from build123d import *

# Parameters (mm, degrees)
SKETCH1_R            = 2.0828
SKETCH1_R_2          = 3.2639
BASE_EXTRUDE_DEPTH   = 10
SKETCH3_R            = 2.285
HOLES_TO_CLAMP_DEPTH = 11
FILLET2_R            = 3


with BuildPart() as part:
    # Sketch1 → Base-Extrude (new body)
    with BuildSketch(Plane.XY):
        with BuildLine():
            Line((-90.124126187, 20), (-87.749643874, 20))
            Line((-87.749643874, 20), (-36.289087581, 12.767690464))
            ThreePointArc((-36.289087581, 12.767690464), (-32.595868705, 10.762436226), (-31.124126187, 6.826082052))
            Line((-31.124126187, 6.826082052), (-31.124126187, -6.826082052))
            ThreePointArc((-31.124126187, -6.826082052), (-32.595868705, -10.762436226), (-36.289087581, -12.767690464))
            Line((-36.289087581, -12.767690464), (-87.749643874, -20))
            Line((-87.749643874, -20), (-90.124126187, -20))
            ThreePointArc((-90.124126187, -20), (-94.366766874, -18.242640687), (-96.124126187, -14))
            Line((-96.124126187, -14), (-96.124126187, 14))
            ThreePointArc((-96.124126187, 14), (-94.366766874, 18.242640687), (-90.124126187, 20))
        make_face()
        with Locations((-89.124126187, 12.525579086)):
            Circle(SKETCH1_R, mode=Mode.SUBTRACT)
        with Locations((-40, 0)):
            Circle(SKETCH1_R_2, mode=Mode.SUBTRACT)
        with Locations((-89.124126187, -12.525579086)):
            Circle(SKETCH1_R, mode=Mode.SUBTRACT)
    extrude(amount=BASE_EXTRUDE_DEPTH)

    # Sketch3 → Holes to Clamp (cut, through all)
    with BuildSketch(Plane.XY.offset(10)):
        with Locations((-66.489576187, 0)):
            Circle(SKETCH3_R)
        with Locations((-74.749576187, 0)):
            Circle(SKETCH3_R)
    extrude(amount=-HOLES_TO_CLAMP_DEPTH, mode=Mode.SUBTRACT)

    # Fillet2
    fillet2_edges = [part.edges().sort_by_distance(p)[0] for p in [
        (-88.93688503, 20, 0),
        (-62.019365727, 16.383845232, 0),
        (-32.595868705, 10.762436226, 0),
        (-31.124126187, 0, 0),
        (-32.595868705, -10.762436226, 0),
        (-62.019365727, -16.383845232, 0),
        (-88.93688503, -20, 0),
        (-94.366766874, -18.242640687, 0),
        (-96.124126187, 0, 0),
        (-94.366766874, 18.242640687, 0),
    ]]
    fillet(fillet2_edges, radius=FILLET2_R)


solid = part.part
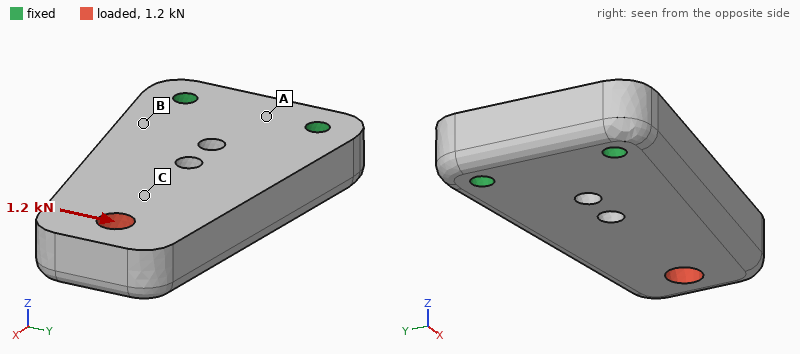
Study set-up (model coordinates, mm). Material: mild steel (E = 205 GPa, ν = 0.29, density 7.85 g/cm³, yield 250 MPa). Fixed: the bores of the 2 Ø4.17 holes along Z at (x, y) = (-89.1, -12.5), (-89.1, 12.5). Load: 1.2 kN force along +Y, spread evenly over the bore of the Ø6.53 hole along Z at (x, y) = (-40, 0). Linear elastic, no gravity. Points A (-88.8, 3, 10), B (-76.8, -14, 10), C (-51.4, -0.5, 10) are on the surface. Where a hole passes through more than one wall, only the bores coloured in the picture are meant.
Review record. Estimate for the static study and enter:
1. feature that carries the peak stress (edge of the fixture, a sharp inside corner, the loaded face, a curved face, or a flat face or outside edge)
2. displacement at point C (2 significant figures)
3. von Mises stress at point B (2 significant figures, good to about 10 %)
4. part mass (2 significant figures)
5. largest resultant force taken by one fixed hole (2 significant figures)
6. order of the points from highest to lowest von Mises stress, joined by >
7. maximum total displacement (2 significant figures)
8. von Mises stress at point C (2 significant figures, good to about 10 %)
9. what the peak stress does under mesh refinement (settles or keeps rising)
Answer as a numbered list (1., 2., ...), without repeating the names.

1. edge of the fixture
2. 6.0 µm
3. 16 MPa
4. 160 g
5. 2.2 kN
6. B > C > A
7. 11 µm
8. 11 MPa
9. keeps rising
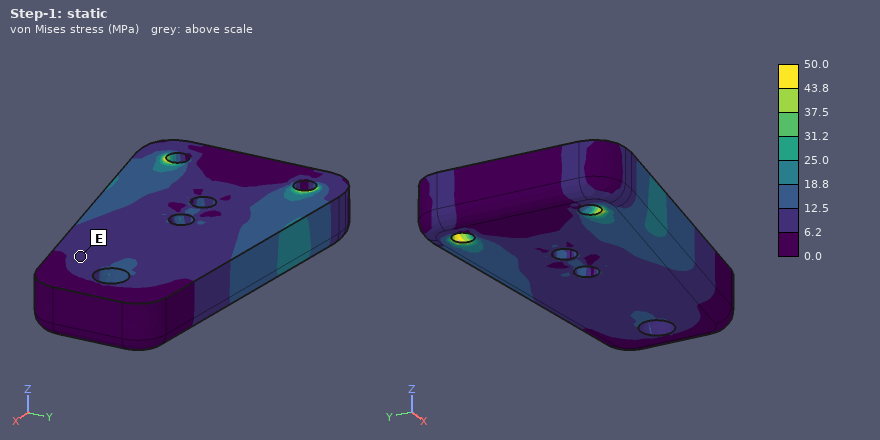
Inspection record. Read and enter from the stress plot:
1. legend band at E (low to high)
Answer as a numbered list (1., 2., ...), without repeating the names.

1. 6.2 to 12.5 MPa
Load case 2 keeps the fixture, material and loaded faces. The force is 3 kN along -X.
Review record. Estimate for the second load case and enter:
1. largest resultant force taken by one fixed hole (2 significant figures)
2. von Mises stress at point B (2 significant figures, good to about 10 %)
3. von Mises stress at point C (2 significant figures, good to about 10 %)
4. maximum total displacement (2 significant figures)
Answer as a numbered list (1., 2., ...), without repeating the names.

1. 1.5 kN
2. 9.4 MPa
3. 12 MPa
4. 3.6 µm
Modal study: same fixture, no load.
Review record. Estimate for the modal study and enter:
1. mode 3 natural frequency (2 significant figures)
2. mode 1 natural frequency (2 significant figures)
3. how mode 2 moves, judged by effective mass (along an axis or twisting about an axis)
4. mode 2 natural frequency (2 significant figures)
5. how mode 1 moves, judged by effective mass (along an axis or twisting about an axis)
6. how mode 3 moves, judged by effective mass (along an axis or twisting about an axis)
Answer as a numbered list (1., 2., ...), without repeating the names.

1. 10 kHz
2. 2700 Hz
3. along Y
4. 8300 Hz
5. along Z
6. twisting about X
